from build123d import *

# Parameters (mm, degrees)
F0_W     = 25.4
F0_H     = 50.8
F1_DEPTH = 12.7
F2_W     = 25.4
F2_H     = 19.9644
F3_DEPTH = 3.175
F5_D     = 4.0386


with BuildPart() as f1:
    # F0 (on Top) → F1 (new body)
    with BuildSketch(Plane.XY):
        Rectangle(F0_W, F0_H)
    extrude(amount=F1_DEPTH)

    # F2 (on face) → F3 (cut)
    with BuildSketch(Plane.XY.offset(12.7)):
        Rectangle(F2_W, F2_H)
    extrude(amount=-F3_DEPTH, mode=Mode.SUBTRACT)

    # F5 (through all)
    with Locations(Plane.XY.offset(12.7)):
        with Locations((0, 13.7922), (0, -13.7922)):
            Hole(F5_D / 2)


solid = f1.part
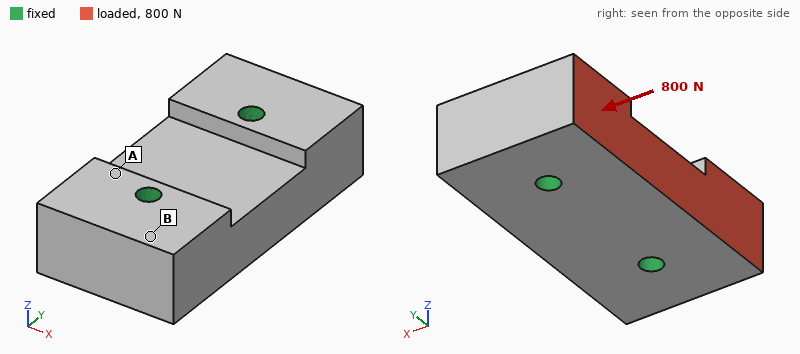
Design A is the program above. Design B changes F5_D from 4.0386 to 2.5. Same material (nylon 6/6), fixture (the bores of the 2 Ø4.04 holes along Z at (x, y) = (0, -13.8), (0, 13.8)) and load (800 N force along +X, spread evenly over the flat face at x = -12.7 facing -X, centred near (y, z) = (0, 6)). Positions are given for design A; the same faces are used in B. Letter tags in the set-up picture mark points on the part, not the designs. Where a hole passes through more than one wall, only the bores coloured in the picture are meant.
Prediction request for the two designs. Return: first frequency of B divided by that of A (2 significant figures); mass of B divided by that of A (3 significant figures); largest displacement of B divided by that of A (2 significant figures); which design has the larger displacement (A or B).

0.83
1.01
1.1
B
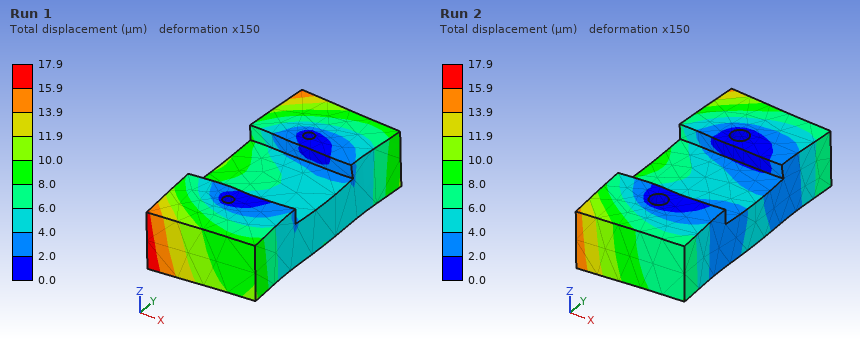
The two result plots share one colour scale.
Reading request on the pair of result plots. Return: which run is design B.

Run 1
